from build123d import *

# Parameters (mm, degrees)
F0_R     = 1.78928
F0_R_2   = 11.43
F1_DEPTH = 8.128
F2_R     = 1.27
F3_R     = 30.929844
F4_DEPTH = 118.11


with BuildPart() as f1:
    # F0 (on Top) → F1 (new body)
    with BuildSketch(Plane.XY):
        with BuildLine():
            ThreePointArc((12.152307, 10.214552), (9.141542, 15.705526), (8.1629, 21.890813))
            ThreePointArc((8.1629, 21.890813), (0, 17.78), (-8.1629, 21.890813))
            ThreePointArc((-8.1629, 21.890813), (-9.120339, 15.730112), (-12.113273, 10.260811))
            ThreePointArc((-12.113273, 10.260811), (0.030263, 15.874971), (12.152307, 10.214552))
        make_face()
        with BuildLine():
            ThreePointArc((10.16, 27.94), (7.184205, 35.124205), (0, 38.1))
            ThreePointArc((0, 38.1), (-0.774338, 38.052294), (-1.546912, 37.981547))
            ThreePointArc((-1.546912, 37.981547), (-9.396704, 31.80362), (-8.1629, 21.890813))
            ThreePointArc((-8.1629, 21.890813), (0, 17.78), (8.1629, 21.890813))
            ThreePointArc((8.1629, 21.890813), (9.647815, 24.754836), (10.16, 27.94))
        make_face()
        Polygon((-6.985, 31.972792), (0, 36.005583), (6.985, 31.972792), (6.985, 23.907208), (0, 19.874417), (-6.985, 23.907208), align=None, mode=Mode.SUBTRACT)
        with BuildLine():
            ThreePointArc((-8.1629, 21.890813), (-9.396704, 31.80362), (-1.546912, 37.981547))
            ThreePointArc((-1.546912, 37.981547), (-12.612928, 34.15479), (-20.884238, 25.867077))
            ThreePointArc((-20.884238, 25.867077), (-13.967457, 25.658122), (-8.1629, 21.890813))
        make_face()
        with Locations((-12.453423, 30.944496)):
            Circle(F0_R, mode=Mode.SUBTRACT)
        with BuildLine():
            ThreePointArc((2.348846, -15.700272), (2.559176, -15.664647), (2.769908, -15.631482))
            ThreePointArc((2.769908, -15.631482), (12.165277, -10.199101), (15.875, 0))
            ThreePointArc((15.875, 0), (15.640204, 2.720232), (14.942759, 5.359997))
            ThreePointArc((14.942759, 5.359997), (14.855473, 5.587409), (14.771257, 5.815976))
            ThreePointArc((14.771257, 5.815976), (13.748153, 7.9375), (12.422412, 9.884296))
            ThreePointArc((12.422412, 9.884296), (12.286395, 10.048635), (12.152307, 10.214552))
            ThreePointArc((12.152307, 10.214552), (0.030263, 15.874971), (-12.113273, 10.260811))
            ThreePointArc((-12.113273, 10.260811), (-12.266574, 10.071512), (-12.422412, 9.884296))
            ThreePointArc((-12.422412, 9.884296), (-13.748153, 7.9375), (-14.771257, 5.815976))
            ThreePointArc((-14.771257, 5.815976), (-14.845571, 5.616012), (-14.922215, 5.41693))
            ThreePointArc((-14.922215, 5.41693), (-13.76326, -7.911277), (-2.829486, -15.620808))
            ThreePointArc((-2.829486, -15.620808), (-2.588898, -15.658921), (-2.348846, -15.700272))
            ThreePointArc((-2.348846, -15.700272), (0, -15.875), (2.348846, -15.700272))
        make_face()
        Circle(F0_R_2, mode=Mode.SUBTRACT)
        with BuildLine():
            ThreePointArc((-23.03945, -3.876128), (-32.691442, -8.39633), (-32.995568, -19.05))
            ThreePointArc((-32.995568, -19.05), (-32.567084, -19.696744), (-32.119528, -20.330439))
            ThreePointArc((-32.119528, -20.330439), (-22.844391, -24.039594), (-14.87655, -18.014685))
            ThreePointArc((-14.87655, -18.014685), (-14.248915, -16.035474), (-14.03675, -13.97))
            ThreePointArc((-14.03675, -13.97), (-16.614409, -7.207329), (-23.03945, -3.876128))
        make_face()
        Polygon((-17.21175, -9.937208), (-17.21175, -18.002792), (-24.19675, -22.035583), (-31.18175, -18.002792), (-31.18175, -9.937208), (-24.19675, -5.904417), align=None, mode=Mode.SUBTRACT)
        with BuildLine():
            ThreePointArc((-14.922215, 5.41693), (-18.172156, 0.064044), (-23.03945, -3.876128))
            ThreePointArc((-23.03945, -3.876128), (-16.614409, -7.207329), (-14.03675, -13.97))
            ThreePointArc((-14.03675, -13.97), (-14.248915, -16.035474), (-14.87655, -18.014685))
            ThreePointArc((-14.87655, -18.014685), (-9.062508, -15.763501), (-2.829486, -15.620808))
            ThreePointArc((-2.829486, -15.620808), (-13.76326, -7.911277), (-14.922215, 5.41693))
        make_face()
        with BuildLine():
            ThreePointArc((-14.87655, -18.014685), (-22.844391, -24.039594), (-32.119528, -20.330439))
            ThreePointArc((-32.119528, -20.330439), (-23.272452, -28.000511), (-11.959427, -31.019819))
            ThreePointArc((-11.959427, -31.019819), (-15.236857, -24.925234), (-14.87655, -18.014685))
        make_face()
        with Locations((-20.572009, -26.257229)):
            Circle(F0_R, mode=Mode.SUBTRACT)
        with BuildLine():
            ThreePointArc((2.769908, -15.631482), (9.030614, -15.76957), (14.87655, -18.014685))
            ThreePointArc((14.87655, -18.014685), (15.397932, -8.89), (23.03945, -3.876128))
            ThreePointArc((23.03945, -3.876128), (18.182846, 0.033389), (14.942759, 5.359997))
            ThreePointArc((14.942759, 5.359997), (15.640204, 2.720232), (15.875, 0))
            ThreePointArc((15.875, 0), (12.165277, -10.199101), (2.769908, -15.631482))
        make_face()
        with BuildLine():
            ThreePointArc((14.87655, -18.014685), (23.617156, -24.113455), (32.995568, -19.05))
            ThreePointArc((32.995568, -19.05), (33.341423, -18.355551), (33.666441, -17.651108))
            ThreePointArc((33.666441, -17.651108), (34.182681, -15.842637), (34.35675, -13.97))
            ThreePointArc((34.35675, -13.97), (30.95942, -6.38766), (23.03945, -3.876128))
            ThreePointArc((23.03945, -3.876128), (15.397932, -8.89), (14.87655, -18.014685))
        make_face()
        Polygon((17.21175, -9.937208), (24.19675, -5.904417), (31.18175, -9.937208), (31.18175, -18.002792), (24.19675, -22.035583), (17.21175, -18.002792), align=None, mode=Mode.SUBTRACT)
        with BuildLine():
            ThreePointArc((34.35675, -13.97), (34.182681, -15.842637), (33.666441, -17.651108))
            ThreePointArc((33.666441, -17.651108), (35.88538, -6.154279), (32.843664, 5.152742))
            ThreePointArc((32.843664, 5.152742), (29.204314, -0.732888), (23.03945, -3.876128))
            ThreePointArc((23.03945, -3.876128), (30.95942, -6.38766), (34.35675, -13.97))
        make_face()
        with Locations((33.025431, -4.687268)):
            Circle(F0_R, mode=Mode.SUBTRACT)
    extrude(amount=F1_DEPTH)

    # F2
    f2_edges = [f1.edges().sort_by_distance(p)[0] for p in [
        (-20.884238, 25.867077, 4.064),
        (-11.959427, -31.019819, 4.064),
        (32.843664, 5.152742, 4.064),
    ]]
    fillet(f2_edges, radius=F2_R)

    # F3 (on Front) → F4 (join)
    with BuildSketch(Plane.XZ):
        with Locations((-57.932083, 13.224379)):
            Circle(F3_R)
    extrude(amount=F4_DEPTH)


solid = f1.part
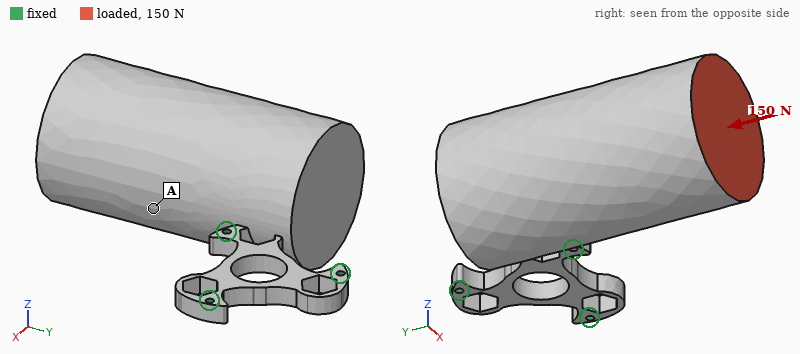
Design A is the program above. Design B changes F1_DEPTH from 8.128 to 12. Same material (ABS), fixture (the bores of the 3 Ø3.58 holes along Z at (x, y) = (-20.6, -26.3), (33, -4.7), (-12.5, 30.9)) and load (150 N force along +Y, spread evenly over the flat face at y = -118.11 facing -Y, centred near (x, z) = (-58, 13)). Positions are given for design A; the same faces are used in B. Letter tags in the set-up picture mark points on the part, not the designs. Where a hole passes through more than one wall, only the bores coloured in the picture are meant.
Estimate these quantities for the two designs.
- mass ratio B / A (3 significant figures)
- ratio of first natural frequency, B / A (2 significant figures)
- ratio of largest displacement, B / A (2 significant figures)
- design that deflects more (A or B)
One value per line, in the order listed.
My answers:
1.01
1.6
0.56
A
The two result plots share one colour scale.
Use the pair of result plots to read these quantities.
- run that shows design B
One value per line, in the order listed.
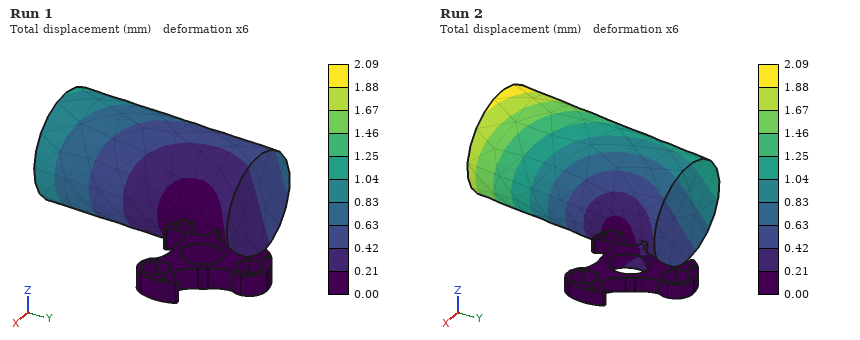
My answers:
Run 1
